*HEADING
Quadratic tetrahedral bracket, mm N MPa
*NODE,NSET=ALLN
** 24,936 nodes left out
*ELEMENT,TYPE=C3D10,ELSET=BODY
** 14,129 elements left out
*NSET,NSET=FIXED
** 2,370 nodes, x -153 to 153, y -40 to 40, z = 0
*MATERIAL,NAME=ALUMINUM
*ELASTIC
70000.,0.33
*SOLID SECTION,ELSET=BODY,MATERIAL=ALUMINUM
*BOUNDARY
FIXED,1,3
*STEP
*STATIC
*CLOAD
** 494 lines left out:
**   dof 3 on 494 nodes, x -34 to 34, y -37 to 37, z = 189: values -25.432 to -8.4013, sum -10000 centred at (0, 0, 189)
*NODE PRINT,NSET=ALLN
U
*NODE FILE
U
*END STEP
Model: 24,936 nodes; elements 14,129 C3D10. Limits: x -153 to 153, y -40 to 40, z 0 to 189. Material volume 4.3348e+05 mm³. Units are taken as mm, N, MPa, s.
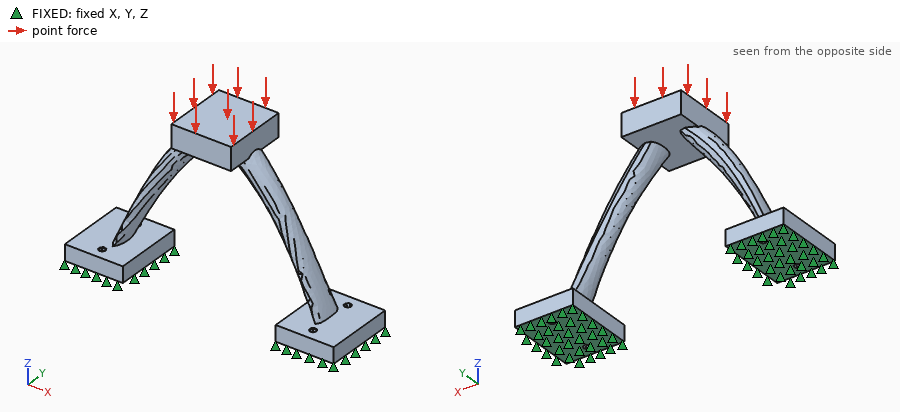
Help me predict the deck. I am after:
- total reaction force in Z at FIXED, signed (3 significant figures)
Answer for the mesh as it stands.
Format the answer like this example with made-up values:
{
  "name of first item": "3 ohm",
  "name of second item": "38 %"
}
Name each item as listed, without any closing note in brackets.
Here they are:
{
  "total reaction force in Z at FIXED, signed": "10000 N"
}
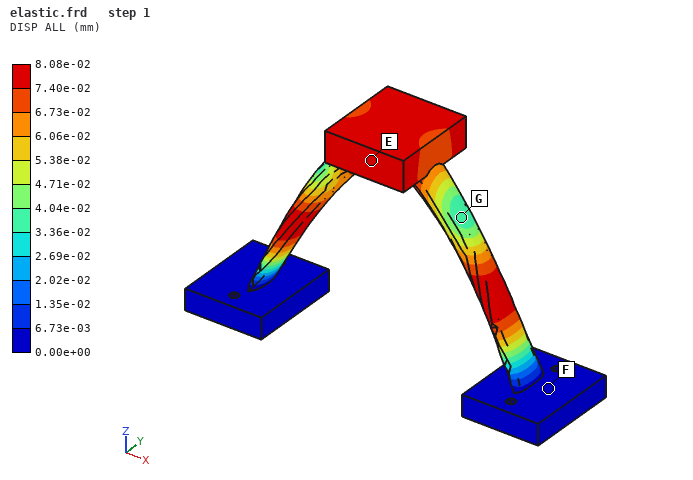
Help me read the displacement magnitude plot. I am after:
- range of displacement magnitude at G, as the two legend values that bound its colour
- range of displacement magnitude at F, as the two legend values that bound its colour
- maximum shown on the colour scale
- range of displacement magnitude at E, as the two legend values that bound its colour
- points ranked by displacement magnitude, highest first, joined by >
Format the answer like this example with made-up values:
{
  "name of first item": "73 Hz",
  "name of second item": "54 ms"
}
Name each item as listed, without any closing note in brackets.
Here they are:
{
  "range of displacement magnitude at G, as the two legend values that bound its colour": "3.36e-02 to 4.04e-02 mm",
  "range of displacement magnitude at F, as the two legend values that bound its colour": "0.00e+00 to 6.73e-03 mm",
  "maximum shown on the colour scale": "8.08e-02 mm",
  "range of displacement magnitude at E, as the two legend values that bound its colour": "7.40e-02 to 8.08e-02 mm",
  "points ranked by displacement magnitude, highest first, joined by >": "E > G > F"
}
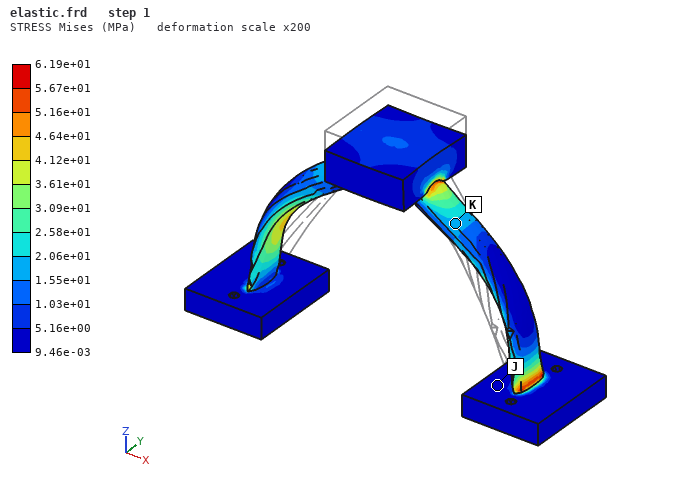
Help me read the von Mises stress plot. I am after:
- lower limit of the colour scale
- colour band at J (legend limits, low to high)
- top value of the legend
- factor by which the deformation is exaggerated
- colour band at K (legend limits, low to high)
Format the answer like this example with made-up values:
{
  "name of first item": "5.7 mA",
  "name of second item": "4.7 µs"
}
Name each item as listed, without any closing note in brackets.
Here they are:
{
  "lower limit of the colour scale": "9.46e-03 MPa",
  "colour band at J": "9.46e-03 to 5.16e+00 MPa",
  "top value of the legend": "6.19e+01 MPa",
  "factor by which the deformation is exaggerated": "200",
  "colour band at K": "1.55e+01 to 2.06e+01 MPa"
}
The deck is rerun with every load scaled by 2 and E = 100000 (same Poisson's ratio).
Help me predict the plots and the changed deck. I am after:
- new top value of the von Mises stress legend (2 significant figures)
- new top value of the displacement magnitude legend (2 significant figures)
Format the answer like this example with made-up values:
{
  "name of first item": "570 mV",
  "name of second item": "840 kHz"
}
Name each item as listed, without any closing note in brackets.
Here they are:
{
  "new top value of the von Mises stress legend": "120 MPa",
  "new top value of the displacement magnitude legend": "0.11 mm"
}
